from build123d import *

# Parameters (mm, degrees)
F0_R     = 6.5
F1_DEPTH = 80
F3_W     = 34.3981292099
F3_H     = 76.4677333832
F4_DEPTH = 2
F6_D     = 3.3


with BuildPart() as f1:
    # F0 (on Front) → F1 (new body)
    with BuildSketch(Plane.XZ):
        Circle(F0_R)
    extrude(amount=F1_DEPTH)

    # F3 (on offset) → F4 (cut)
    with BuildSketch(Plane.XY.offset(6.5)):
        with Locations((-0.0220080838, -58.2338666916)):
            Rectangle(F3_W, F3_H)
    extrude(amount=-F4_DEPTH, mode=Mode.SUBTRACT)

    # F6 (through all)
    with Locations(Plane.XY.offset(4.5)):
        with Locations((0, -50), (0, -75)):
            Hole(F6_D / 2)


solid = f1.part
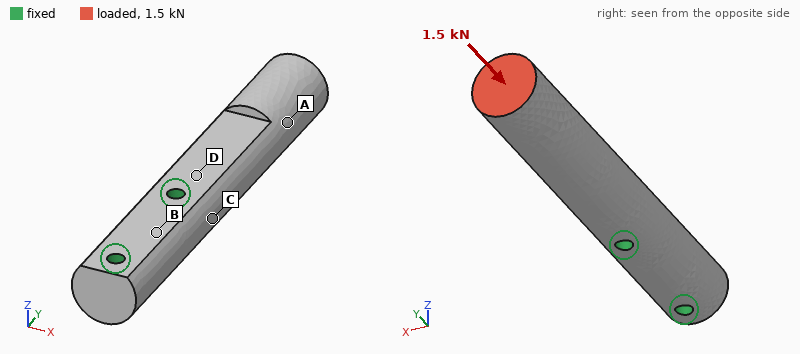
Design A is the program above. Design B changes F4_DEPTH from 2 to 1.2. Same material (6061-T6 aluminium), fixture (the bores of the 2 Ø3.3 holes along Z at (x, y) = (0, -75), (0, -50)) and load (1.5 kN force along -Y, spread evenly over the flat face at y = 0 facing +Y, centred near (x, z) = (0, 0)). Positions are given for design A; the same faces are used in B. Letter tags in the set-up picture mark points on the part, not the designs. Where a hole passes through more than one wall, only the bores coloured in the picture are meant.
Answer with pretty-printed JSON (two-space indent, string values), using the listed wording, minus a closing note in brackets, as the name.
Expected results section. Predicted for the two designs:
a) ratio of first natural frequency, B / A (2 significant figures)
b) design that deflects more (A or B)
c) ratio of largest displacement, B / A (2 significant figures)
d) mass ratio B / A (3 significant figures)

{
  "ratio of first natural frequency, B / A": "1.0",
  "design that deflects more": "A",
  "ratio of largest displacement, B / A": "0.61",
  "mass ratio B / A": "1.04"
}
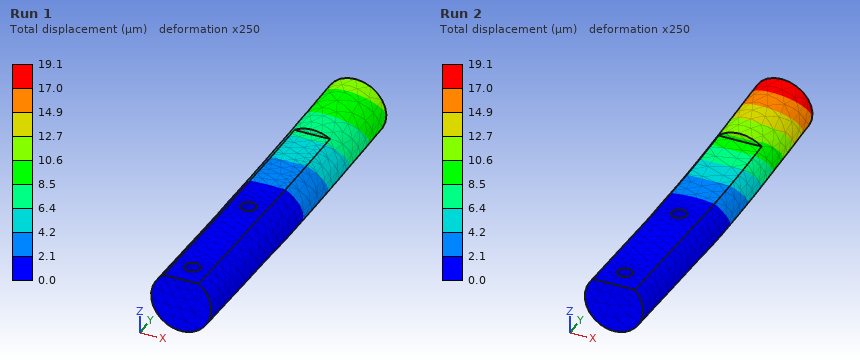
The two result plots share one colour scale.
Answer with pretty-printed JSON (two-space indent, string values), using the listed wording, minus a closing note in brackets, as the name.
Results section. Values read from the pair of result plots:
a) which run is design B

{
  "which run is design B": "Run 1"
}
